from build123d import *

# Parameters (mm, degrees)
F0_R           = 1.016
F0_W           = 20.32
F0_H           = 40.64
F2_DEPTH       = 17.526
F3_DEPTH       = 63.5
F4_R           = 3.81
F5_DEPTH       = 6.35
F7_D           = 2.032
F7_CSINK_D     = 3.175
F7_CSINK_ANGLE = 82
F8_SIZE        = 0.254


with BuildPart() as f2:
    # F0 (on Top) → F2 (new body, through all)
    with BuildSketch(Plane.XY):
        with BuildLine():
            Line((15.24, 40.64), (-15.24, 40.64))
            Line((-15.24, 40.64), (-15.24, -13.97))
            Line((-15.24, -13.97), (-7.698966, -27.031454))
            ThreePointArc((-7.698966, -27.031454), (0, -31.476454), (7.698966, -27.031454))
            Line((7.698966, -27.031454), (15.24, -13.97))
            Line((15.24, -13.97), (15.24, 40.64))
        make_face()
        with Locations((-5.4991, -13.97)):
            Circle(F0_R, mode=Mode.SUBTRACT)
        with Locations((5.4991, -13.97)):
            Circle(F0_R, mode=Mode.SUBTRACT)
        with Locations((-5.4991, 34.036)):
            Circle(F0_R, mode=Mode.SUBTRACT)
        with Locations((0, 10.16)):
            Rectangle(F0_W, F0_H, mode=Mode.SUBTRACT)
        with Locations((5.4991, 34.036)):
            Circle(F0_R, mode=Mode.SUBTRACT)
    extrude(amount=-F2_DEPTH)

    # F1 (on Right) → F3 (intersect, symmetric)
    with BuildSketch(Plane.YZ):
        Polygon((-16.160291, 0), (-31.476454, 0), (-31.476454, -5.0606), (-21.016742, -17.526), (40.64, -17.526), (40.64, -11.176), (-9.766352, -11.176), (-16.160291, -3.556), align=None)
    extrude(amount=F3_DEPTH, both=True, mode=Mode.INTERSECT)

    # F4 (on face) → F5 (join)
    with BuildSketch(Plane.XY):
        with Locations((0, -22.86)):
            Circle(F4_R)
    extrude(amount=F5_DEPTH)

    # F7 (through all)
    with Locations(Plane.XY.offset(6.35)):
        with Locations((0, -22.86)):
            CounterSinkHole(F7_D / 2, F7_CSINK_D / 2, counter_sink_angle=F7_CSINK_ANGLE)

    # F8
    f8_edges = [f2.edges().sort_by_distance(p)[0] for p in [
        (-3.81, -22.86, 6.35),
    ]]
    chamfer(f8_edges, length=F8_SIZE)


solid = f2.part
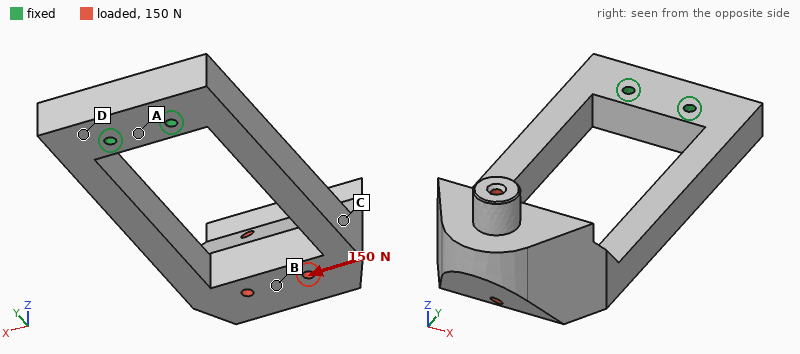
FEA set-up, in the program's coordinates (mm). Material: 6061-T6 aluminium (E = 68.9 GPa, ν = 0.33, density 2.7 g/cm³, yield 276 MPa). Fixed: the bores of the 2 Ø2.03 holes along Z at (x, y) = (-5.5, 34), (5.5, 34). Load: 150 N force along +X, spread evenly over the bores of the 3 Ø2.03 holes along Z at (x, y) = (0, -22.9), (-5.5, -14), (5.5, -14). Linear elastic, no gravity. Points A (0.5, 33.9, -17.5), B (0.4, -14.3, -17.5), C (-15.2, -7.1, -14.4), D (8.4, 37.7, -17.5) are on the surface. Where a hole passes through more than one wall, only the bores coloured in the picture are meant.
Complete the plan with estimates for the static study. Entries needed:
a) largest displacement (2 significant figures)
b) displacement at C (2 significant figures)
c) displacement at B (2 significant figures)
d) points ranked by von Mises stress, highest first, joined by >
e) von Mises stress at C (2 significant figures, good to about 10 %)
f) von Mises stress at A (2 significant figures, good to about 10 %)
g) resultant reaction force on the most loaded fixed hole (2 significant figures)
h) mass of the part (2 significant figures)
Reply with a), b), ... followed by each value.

a) 0.22 mm
b) 0.16 mm
c) 0.16 mm
d) C > D > A > B
e) 42 MPa
f) 11 MPa
g) 560 N
h) 29 g
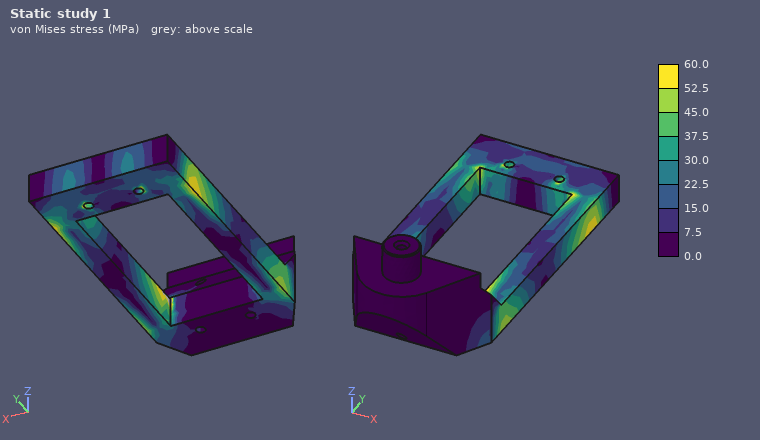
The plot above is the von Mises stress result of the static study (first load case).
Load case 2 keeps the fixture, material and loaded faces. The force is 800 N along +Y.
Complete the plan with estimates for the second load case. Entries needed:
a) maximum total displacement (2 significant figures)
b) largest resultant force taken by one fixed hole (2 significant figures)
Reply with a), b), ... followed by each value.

a) 0.73 mm
b) 450 N
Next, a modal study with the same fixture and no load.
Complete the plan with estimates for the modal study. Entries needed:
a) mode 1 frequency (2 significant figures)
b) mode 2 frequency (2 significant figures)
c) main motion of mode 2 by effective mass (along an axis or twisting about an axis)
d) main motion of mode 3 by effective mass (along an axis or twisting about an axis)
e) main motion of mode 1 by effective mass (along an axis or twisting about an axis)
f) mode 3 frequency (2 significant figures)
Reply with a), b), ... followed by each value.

a) 580 Hz
b) 1000 Hz
c) along X
d) twisting about Y
e) along Z
f) 2400 Hz
